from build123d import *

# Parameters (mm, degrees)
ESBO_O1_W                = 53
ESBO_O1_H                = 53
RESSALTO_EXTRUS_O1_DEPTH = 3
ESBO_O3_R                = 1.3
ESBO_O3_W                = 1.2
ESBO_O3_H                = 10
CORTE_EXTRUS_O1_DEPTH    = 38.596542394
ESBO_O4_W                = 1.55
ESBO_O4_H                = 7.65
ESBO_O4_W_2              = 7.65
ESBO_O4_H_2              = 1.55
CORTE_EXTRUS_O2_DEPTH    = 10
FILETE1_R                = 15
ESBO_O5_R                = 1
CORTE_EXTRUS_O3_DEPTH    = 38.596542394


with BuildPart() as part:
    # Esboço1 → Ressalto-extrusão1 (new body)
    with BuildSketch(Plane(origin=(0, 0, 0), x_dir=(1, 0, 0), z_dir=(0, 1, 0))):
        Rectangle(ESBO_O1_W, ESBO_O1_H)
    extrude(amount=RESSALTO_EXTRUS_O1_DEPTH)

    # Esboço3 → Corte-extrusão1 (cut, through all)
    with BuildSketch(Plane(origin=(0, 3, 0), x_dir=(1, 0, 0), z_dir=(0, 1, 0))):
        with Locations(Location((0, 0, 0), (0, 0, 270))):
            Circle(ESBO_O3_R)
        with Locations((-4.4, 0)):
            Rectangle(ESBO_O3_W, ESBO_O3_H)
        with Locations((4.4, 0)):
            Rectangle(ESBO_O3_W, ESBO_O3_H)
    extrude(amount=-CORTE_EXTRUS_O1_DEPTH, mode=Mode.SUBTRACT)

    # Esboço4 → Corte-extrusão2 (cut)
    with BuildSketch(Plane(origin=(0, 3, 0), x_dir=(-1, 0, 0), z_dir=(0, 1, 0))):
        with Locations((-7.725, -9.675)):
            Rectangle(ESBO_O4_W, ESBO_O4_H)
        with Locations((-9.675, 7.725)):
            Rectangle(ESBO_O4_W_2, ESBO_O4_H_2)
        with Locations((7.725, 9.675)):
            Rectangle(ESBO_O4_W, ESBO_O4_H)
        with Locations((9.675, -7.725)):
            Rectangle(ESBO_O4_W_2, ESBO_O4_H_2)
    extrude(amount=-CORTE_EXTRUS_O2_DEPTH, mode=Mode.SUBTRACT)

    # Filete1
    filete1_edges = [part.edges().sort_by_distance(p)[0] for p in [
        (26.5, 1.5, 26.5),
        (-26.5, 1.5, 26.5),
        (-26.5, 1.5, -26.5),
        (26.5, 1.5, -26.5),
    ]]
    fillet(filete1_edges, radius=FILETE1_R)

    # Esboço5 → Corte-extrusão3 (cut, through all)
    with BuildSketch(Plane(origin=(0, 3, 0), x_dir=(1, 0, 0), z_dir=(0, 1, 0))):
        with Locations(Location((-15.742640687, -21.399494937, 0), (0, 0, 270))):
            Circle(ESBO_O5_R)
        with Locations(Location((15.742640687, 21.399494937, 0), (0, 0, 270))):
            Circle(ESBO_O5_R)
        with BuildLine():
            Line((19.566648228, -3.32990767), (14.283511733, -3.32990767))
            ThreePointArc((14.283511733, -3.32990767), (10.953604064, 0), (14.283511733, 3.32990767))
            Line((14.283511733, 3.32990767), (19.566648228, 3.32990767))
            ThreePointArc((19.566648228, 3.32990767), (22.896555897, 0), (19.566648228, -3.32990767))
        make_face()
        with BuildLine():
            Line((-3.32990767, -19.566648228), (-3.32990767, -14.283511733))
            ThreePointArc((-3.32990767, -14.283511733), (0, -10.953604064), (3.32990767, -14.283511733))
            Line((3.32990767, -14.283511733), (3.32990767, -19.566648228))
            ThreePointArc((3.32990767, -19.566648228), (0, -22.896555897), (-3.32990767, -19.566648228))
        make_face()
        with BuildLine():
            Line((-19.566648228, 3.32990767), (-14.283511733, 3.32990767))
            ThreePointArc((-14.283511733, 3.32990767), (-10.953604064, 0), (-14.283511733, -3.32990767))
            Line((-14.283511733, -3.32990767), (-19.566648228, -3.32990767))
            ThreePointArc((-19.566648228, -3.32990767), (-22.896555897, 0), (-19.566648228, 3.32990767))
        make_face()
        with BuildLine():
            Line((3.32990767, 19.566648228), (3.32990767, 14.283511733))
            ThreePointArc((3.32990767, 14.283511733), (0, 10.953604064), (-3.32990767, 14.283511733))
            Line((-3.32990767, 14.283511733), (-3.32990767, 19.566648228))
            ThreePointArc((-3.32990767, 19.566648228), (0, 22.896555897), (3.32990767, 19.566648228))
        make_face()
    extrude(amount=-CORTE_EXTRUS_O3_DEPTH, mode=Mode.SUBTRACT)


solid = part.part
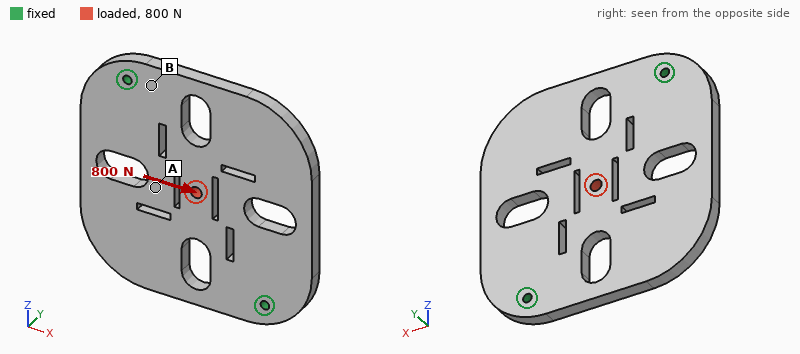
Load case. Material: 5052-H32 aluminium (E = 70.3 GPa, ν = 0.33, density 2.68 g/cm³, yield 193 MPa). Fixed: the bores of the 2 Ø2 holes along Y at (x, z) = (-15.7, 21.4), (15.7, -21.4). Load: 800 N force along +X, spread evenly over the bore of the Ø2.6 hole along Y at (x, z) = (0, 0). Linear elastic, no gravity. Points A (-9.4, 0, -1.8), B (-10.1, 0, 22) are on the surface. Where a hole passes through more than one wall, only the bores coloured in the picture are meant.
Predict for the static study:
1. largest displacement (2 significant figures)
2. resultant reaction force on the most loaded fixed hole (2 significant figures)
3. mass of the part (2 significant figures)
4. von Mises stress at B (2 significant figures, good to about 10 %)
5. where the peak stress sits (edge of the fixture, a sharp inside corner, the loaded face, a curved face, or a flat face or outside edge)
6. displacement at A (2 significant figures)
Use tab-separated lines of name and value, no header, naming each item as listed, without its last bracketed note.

largest displacement	14 µm
resultant reaction force on the most loaded fixed hole	400 N
mass of the part	18 g
von Mises stress at B	11 MPa
where the peak stress sits	a sharp inside corner
displacement at A	6.2 µm
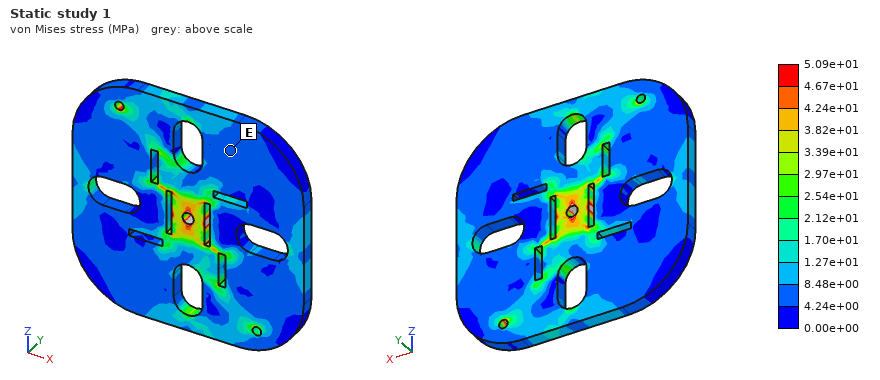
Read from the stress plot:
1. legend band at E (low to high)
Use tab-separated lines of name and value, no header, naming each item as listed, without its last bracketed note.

legend band at E	4.24e+00 to 8.48e+00 MPa
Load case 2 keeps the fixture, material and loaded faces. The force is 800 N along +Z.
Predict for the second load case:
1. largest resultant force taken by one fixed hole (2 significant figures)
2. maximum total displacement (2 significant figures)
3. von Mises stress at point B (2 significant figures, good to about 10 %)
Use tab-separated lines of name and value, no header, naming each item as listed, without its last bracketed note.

largest resultant force taken by one fixed hole	400 N
maximum total displacement	8.1 µm
von Mises stress at point B	8.1 MPa
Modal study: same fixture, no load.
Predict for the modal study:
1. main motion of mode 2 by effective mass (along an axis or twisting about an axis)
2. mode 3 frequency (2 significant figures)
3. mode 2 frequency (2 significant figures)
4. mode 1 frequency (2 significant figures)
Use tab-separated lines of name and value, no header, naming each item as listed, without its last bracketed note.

main motion of mode 2 by effective mass	along Y
mode 3 frequency	6000 Hz
mode 2 frequency	2600 Hz
mode 1 frequency	1900 Hz
